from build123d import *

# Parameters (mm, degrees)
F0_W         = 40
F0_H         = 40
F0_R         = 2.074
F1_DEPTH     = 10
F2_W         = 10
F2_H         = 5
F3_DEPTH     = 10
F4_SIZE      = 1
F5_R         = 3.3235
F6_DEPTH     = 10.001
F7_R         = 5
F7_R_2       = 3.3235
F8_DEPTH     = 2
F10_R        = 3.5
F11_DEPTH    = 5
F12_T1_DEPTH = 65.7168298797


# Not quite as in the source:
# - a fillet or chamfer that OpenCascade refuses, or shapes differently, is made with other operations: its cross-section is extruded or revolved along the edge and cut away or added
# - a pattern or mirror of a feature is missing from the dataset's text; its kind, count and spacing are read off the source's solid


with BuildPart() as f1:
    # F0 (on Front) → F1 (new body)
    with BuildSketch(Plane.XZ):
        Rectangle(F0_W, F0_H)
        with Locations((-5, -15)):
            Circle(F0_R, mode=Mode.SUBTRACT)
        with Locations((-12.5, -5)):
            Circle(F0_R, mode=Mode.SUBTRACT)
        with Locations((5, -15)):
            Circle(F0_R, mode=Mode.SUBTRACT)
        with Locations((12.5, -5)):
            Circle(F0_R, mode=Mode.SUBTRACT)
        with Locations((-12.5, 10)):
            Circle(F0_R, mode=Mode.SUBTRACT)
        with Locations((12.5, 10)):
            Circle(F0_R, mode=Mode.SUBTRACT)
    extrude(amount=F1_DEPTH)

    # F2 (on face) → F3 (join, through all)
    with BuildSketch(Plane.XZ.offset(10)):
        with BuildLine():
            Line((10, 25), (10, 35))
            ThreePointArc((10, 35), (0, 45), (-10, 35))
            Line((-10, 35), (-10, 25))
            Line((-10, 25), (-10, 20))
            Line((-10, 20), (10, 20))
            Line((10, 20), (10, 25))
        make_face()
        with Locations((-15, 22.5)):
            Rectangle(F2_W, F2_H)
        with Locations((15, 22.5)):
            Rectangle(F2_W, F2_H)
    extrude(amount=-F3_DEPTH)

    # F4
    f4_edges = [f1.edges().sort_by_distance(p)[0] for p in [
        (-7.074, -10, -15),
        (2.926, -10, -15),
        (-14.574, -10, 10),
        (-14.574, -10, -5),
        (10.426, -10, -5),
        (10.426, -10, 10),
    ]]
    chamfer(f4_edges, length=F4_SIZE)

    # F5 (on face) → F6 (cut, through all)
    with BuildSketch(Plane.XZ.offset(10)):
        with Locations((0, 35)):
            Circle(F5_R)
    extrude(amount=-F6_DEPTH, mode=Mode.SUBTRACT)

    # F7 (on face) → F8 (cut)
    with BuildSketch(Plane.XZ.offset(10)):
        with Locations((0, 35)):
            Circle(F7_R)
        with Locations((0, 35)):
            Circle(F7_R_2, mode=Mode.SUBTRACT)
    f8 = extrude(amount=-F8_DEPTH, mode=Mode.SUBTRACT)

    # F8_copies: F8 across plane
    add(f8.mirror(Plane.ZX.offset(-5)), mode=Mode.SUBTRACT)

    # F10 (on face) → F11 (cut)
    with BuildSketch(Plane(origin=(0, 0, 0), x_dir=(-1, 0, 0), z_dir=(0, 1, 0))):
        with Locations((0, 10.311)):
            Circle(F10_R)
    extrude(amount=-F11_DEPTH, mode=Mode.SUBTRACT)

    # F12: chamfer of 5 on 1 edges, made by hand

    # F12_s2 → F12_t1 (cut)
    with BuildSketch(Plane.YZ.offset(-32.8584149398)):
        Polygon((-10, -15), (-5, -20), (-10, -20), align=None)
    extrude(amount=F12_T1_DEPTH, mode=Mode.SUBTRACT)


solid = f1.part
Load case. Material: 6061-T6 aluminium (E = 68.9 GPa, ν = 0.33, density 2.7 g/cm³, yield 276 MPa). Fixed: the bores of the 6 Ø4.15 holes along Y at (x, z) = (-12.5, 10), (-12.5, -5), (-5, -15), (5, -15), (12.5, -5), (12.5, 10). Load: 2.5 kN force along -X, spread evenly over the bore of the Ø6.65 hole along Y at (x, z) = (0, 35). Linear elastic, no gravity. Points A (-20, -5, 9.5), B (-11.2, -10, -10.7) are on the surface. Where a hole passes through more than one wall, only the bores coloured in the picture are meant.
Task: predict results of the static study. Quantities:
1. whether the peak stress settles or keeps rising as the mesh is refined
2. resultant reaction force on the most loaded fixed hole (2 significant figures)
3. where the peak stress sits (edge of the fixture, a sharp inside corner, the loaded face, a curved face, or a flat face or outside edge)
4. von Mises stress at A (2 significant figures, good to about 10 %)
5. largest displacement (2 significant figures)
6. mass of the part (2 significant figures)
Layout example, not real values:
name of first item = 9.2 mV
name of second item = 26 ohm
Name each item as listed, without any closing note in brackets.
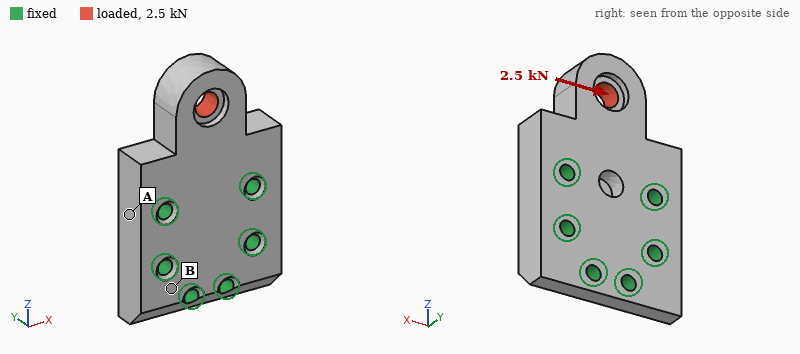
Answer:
whether the peak stress settles or keeps rising as the mesh is refined = keeps rising
resultant reaction force on the most loaded fixed hole = 2.3 kN
where the peak stress sits = edge of the fixture
von Mises stress at A = 16 MPa
largest displacement = 30 µm
mass of the part = 53 g
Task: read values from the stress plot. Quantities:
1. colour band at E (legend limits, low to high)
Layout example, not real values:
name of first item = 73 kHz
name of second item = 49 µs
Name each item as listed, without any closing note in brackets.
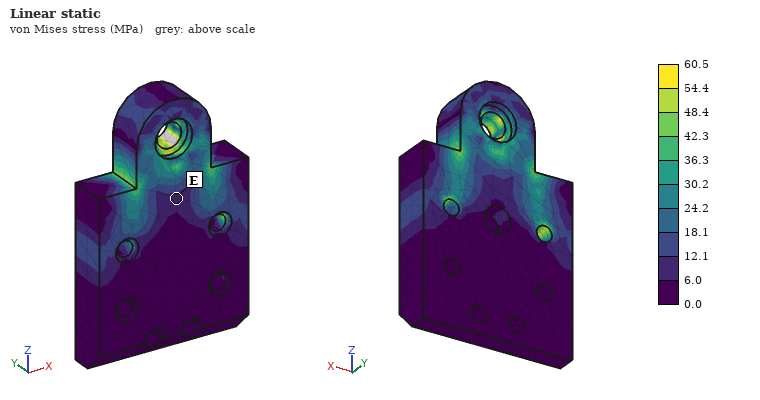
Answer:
colour band at E = 6.0 to 12.1 MPa
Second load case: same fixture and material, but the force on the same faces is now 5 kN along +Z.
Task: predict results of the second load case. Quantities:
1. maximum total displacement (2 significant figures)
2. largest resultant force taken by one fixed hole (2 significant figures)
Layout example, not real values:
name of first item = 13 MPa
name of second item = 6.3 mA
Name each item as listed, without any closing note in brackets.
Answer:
maximum total displacement = 14 µm
largest resultant force taken by one fixed hole = 2.1 kN
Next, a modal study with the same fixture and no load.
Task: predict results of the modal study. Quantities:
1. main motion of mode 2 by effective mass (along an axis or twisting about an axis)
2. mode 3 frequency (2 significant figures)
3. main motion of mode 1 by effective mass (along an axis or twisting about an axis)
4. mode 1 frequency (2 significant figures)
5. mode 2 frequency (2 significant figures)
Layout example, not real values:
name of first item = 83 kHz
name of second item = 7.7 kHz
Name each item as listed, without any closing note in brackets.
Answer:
main motion of mode 2 by effective mass = along X
mode 3 frequency = 23 kHz
main motion of mode 1 by effective mass = along Y
mode 1 frequency = 8200 Hz
mode 2 frequency = 19 kHz
